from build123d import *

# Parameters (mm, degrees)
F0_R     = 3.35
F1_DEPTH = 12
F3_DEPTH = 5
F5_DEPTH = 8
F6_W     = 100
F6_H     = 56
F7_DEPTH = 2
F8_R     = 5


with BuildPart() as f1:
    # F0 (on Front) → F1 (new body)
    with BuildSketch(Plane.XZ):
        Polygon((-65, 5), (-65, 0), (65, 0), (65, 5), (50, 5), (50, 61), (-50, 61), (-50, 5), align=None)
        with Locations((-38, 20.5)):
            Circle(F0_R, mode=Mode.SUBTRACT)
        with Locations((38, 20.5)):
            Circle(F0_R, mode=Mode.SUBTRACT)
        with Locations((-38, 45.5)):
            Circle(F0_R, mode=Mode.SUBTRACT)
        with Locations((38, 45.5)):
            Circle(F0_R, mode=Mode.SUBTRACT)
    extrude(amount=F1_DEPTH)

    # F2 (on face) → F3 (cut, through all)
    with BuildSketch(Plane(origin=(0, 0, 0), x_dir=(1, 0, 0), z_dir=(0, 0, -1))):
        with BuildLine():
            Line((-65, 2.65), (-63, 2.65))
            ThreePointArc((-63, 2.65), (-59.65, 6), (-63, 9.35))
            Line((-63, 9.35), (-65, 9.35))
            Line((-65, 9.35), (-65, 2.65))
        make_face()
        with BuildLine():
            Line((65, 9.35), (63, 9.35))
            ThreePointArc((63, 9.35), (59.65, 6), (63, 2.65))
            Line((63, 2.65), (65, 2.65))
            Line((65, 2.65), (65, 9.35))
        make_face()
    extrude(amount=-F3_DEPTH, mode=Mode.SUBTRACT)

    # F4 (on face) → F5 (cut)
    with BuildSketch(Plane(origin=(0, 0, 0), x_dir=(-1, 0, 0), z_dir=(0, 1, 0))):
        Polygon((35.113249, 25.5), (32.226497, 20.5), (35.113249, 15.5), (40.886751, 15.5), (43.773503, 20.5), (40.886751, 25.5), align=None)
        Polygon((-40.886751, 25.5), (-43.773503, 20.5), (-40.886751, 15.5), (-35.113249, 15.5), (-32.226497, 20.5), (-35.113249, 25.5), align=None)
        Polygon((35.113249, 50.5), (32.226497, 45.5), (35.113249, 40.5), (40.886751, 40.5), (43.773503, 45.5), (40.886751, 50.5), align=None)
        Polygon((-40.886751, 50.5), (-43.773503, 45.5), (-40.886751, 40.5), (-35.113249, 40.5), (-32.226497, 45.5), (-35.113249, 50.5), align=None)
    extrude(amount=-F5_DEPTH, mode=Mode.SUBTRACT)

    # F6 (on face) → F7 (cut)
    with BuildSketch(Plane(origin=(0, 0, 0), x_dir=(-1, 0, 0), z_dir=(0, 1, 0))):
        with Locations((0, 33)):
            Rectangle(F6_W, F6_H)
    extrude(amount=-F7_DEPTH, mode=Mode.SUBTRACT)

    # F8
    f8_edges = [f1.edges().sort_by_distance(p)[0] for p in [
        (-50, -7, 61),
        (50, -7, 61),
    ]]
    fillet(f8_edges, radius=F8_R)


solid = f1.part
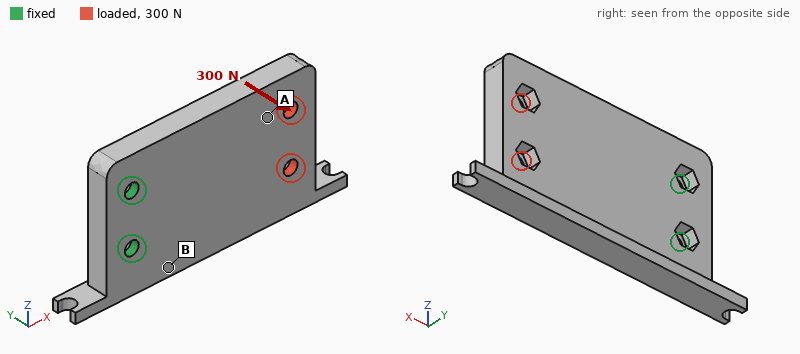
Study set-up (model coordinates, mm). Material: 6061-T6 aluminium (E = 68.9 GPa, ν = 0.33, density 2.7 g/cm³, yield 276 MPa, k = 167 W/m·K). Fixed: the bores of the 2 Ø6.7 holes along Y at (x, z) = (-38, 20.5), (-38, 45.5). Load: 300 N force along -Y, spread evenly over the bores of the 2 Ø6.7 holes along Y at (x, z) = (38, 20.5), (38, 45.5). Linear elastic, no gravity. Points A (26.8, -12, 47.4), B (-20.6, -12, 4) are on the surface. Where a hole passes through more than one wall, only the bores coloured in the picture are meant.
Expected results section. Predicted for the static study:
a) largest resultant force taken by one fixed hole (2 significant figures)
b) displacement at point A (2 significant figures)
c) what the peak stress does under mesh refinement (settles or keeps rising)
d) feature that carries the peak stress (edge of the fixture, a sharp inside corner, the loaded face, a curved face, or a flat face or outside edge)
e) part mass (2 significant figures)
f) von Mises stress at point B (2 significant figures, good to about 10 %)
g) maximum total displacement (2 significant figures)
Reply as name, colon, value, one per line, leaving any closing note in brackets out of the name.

largest resultant force taken by one fixed hole: 240 N
displacement at point A: 0.18 mm
what the peak stress does under mesh refinement: keeps rising
feature that carries the peak stress: edge of the fixture
part mass: 160 g
von Mises stress at point B: 15 MPa
maximum total displacement: 0.32 mm
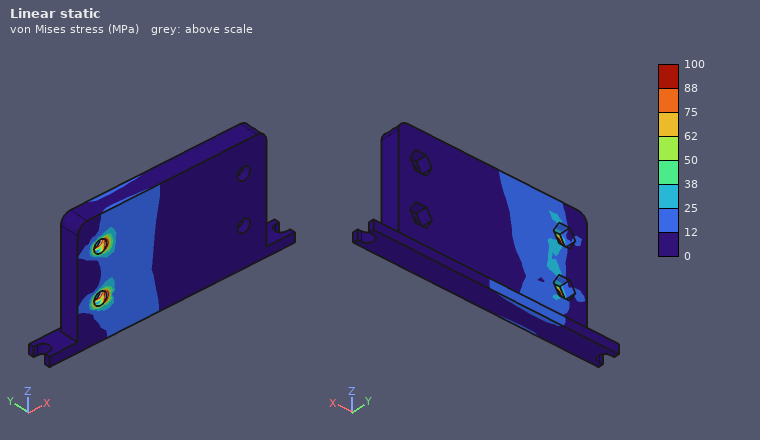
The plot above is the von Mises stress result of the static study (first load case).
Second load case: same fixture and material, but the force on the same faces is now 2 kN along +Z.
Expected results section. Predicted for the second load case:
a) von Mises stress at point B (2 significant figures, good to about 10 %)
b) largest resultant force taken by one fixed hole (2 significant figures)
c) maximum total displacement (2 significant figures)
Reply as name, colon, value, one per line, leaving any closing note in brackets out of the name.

von Mises stress at point B: 17 MPa
largest resultant force taken by one fixed hole: 5.2 kN
maximum total displacement: 0.13 mm
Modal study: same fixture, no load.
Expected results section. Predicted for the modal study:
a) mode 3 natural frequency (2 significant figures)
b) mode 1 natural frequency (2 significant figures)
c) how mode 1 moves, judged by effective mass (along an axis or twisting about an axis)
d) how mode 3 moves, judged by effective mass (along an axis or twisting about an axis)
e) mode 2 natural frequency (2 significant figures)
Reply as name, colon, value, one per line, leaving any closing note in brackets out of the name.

mode 3 natural frequency: 3100 Hz
mode 1 natural frequency: 760 Hz
how mode 1 moves, judged by effective mass: along Y
how mode 3 moves, judged by effective mass: along Z
mode 2 natural frequency: 2600 Hz
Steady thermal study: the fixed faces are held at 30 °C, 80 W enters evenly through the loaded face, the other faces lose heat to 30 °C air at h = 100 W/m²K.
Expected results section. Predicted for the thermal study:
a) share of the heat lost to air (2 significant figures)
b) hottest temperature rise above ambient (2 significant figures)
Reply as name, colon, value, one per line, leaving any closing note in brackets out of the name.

share of the heat lost to air: 47 %
hottest temperature rise above ambient: 53 K
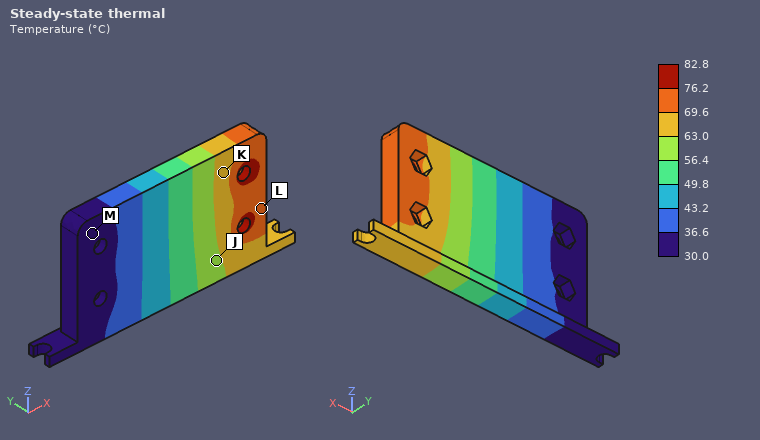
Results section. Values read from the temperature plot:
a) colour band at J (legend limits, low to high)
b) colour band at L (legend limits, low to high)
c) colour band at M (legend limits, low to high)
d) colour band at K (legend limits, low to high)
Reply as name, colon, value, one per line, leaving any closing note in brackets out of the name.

colour band at J: 56.4 to 63.0 °C
colour band at L: 69.6 to 76.2 °C
colour band at M: 30.0 to 36.6 °C
colour band at K: 63.0 to 69.6 °C
